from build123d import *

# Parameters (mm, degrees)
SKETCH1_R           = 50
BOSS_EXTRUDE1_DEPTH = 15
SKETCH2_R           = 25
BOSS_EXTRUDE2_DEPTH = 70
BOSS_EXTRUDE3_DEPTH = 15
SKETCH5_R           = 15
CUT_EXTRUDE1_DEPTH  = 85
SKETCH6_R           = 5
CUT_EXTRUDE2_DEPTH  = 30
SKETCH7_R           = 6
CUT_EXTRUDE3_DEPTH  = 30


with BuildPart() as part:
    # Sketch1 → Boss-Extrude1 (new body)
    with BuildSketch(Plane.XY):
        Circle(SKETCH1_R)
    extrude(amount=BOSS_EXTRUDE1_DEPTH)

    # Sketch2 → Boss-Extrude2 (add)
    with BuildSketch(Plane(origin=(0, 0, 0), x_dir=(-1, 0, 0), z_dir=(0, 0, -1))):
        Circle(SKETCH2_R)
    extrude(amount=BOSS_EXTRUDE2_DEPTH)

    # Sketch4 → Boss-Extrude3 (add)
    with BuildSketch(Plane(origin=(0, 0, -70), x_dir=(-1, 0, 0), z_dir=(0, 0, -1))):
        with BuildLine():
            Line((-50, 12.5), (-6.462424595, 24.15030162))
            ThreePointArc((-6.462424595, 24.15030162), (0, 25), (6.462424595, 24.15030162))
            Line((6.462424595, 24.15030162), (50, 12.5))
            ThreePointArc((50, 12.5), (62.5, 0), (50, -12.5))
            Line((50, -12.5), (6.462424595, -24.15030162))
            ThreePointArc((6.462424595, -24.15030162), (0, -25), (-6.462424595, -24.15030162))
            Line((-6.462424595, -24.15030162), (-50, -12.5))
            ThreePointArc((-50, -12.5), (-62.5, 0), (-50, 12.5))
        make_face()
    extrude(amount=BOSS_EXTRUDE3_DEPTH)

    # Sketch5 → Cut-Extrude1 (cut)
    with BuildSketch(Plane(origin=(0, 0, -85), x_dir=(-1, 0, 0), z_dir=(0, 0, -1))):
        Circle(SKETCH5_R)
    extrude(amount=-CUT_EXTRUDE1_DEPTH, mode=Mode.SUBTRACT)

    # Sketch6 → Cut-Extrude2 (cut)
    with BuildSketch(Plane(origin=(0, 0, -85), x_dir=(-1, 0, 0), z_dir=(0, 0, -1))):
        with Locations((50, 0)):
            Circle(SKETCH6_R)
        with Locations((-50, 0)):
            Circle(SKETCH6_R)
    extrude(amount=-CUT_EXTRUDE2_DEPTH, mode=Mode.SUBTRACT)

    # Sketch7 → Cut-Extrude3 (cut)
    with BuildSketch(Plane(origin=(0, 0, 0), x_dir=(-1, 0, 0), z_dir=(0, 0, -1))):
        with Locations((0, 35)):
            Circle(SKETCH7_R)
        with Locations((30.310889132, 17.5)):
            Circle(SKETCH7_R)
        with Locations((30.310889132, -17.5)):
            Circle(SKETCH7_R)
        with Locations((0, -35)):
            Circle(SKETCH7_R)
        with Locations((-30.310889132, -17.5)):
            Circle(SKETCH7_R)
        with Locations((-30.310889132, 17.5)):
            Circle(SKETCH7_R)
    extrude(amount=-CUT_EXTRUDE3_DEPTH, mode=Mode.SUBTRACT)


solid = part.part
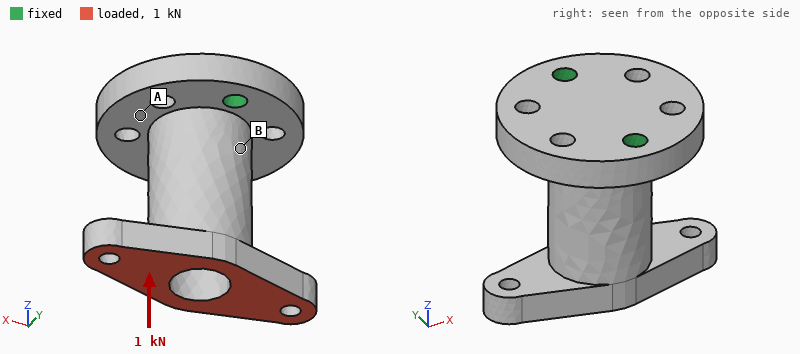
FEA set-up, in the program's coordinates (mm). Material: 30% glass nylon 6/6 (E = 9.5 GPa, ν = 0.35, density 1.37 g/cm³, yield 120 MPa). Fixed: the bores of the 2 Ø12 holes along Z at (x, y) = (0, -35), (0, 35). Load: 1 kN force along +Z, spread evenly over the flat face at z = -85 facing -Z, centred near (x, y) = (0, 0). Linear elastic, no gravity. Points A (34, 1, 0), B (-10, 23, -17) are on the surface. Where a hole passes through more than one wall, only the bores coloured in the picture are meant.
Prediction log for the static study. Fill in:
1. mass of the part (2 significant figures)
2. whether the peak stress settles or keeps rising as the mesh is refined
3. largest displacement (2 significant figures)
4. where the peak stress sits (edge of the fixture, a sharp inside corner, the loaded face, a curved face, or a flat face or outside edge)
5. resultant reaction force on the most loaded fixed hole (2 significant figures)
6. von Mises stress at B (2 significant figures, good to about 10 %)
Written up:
340 g
keeps rising
68 µm
edge of the fixture
510 N
1.1 MPa
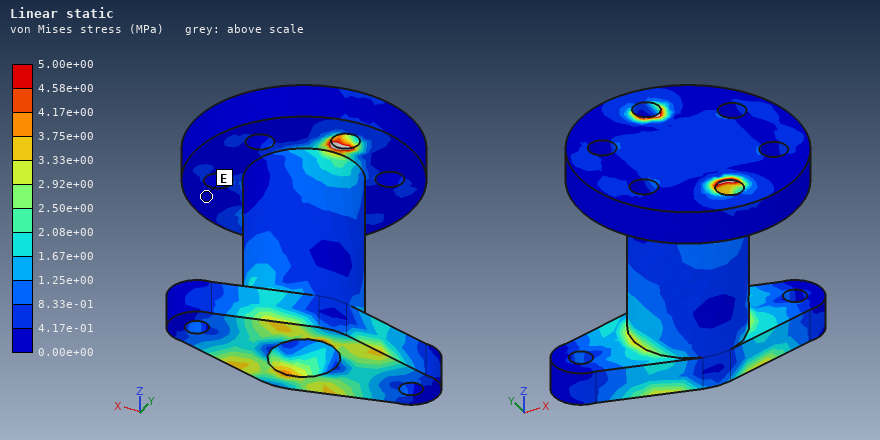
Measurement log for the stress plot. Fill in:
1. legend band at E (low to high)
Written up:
0.00e+00 to 4.17e-01 MPa
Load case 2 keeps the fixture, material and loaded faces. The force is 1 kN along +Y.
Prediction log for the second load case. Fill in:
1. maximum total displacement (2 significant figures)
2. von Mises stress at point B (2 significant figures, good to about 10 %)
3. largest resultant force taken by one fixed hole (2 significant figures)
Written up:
0.18 mm
5.7 MPa
1.7 kN
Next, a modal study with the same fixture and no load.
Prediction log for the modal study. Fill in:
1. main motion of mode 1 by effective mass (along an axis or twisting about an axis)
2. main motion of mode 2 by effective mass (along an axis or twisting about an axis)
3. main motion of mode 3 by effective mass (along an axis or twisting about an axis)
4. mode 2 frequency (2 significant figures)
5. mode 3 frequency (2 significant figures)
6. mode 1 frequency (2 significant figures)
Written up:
along X
along Y
twisting about Z
1300 Hz
2300 Hz
730 Hz
